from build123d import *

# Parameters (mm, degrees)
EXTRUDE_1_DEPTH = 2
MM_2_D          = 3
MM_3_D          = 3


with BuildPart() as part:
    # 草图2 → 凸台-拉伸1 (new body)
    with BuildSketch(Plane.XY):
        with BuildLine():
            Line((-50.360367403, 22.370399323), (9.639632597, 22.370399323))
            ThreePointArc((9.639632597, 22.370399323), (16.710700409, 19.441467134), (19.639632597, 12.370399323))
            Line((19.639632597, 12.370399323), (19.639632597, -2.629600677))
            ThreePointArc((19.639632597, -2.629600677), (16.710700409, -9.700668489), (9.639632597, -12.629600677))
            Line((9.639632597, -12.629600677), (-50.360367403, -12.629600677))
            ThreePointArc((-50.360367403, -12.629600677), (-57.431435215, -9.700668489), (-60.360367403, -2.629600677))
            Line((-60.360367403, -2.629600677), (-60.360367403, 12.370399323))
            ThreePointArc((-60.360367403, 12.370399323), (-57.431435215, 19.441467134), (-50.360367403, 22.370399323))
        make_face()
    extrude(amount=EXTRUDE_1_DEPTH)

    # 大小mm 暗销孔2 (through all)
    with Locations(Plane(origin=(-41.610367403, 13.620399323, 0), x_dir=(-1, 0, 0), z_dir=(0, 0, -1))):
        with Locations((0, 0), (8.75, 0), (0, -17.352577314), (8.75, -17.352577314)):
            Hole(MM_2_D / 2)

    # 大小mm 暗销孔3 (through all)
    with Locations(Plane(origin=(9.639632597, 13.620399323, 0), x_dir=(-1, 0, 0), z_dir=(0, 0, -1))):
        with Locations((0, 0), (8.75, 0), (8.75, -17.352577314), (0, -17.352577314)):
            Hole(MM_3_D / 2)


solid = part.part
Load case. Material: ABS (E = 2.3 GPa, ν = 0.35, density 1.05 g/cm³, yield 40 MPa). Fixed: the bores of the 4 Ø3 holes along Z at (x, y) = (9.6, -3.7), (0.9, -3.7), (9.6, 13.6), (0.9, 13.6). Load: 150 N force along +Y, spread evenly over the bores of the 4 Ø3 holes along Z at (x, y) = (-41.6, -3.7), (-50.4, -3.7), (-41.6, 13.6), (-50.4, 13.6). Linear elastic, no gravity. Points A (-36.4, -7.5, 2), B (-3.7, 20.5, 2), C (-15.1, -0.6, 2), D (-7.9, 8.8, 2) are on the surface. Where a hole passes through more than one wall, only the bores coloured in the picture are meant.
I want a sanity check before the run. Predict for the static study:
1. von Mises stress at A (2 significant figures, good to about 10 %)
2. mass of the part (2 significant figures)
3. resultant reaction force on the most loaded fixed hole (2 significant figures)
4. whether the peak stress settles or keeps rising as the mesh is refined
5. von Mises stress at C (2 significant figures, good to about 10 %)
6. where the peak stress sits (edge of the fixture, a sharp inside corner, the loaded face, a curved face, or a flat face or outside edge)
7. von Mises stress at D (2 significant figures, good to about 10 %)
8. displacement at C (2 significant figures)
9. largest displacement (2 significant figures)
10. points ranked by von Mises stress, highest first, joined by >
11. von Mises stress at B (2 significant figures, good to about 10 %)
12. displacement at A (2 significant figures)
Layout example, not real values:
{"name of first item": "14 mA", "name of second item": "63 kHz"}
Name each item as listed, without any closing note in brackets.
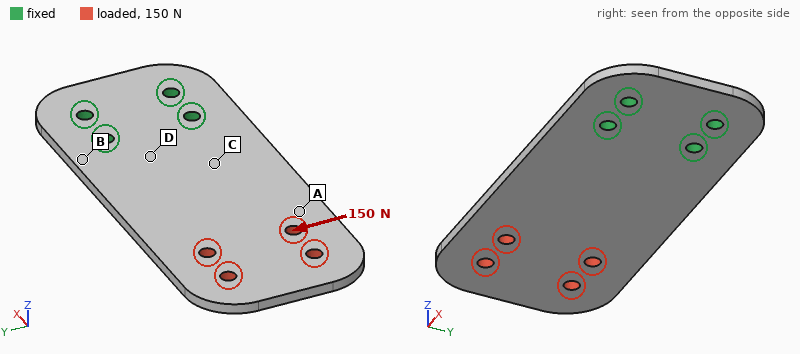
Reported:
{"von Mises stress at A": "3.7 MPa", "mass of the part": "5.6 g", "resultant reaction force on the most loaded fixed hole": "270 N", "whether the peak stress settles or keeps rising as the mesh is refined": "keeps rising", "von Mises stress at C": "6.7 MPa", "where the peak stress sits": "edge of the fixture", "von Mises stress at D": "8.1 MPa", "displacement at C": "0.14 mm", "largest displacement": "0.75 mm", "points ranked by von Mises stress, highest first, joined by >": "B > D > C > A", "von Mises stress at B": "11 MPa", "displacement at A": "0.44 mm"}
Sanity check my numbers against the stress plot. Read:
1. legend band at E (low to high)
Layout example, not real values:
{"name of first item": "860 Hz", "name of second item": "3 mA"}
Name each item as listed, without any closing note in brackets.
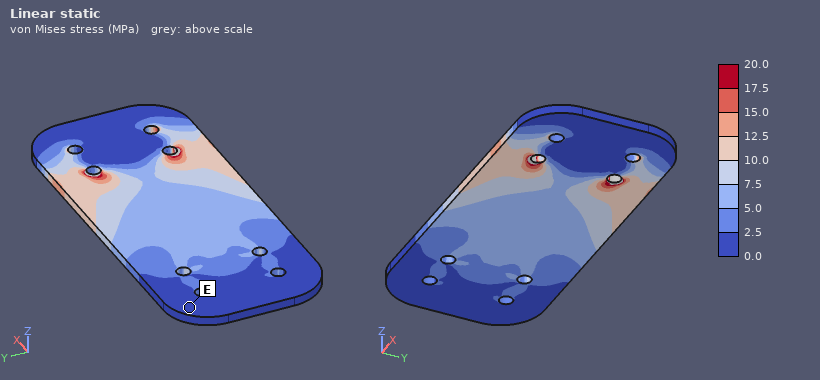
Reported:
{"legend band at E": "0.0 to 2.5 MPa"}
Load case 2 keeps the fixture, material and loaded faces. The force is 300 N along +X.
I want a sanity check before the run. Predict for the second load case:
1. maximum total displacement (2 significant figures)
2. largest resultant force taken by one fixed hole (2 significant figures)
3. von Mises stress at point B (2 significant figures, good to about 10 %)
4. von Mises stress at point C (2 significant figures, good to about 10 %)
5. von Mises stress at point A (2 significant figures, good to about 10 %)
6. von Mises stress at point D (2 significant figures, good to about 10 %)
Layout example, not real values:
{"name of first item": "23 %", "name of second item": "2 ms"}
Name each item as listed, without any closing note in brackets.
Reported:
{"maximum total displacement": "0.10 mm", "largest resultant force taken by one fixed hole": "110 N", "von Mises stress at point B": "3.1 MPa", "von Mises stress at point C": "4.5 MPa", "von Mises stress at point A": "4.5 MPa", "von Mises stress at point D": "4.3 MPa"}
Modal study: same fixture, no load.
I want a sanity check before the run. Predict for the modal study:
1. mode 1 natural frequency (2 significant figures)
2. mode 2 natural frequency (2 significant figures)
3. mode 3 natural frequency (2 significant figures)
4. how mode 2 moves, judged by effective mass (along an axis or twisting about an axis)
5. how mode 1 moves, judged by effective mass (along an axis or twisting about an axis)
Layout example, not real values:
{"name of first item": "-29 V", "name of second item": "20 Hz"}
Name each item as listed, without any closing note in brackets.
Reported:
{"mode 1 natural frequency": "140 Hz", "mode 2 natural frequency": "510 Hz", "mode 3 natural frequency": "830 Hz", "how mode 2 moves, judged by effective mass": "twisting about X", "how mode 1 moves, judged by effective mass": "along Z"}
